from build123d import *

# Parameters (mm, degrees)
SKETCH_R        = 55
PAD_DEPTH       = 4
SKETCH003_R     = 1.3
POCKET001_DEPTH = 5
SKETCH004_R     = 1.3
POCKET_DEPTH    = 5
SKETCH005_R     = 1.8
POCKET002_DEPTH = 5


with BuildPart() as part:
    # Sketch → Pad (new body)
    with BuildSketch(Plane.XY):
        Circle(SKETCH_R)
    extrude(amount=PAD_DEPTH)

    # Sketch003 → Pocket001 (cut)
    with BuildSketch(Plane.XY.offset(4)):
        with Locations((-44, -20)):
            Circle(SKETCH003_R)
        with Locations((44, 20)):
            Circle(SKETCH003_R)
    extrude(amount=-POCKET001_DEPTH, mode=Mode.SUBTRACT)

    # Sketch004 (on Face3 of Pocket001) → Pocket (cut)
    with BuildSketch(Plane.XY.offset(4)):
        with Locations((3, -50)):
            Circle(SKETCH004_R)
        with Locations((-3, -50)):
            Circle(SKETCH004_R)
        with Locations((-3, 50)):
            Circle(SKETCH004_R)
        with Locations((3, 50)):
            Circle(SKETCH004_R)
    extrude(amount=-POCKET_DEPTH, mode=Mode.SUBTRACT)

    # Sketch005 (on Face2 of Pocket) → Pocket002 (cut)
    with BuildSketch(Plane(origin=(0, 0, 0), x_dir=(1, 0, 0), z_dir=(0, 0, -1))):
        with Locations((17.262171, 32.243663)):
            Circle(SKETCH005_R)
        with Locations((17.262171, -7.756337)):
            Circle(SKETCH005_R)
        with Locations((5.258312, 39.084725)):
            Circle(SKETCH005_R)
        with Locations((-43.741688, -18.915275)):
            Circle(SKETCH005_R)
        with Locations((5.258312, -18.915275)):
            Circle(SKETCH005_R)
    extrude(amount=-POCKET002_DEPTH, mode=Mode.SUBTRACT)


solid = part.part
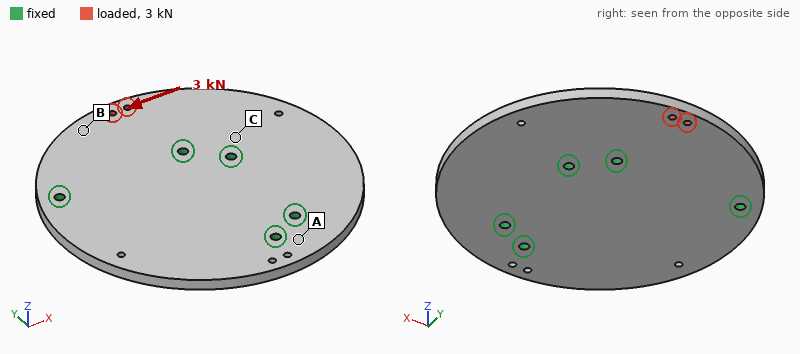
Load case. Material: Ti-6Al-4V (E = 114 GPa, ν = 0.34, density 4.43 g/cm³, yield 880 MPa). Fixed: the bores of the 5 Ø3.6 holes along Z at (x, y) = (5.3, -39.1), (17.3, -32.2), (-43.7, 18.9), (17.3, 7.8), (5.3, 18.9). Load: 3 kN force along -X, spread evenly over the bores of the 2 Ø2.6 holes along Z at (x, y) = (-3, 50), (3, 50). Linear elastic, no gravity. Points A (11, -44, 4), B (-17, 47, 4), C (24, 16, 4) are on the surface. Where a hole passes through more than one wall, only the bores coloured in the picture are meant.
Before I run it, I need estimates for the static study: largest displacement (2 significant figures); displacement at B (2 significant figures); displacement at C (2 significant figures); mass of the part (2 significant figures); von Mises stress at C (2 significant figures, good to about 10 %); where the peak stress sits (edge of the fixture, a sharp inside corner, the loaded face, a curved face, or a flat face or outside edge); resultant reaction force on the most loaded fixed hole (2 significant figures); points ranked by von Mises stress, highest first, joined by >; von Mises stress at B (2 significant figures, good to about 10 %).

16 µm
9.4 µm
2.9 µm
170 g
11 MPa
the loaded face
1.7 kN
B > C > A
26 MPa
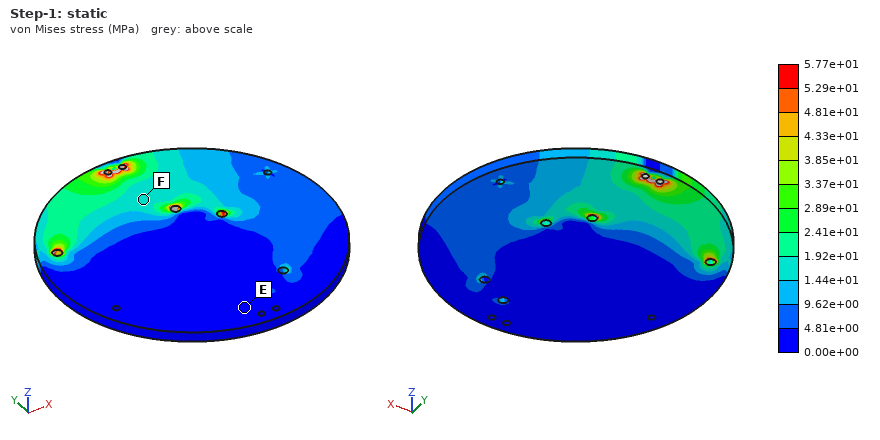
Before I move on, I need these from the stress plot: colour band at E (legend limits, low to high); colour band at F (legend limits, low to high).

0.00e+00 to 4.81e+00 MPa
1.44e+01 to 1.92e+01 MPa
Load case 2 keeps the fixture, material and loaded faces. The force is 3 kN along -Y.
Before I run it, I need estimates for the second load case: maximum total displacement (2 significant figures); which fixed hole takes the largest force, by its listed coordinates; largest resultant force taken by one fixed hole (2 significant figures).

10 µm
(5.3, 18.9)
1.5 kN
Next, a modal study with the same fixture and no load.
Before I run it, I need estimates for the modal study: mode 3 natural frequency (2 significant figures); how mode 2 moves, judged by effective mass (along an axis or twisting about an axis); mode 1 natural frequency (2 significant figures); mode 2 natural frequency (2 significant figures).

2700 Hz
along Z
2200 Hz
2400 Hz
